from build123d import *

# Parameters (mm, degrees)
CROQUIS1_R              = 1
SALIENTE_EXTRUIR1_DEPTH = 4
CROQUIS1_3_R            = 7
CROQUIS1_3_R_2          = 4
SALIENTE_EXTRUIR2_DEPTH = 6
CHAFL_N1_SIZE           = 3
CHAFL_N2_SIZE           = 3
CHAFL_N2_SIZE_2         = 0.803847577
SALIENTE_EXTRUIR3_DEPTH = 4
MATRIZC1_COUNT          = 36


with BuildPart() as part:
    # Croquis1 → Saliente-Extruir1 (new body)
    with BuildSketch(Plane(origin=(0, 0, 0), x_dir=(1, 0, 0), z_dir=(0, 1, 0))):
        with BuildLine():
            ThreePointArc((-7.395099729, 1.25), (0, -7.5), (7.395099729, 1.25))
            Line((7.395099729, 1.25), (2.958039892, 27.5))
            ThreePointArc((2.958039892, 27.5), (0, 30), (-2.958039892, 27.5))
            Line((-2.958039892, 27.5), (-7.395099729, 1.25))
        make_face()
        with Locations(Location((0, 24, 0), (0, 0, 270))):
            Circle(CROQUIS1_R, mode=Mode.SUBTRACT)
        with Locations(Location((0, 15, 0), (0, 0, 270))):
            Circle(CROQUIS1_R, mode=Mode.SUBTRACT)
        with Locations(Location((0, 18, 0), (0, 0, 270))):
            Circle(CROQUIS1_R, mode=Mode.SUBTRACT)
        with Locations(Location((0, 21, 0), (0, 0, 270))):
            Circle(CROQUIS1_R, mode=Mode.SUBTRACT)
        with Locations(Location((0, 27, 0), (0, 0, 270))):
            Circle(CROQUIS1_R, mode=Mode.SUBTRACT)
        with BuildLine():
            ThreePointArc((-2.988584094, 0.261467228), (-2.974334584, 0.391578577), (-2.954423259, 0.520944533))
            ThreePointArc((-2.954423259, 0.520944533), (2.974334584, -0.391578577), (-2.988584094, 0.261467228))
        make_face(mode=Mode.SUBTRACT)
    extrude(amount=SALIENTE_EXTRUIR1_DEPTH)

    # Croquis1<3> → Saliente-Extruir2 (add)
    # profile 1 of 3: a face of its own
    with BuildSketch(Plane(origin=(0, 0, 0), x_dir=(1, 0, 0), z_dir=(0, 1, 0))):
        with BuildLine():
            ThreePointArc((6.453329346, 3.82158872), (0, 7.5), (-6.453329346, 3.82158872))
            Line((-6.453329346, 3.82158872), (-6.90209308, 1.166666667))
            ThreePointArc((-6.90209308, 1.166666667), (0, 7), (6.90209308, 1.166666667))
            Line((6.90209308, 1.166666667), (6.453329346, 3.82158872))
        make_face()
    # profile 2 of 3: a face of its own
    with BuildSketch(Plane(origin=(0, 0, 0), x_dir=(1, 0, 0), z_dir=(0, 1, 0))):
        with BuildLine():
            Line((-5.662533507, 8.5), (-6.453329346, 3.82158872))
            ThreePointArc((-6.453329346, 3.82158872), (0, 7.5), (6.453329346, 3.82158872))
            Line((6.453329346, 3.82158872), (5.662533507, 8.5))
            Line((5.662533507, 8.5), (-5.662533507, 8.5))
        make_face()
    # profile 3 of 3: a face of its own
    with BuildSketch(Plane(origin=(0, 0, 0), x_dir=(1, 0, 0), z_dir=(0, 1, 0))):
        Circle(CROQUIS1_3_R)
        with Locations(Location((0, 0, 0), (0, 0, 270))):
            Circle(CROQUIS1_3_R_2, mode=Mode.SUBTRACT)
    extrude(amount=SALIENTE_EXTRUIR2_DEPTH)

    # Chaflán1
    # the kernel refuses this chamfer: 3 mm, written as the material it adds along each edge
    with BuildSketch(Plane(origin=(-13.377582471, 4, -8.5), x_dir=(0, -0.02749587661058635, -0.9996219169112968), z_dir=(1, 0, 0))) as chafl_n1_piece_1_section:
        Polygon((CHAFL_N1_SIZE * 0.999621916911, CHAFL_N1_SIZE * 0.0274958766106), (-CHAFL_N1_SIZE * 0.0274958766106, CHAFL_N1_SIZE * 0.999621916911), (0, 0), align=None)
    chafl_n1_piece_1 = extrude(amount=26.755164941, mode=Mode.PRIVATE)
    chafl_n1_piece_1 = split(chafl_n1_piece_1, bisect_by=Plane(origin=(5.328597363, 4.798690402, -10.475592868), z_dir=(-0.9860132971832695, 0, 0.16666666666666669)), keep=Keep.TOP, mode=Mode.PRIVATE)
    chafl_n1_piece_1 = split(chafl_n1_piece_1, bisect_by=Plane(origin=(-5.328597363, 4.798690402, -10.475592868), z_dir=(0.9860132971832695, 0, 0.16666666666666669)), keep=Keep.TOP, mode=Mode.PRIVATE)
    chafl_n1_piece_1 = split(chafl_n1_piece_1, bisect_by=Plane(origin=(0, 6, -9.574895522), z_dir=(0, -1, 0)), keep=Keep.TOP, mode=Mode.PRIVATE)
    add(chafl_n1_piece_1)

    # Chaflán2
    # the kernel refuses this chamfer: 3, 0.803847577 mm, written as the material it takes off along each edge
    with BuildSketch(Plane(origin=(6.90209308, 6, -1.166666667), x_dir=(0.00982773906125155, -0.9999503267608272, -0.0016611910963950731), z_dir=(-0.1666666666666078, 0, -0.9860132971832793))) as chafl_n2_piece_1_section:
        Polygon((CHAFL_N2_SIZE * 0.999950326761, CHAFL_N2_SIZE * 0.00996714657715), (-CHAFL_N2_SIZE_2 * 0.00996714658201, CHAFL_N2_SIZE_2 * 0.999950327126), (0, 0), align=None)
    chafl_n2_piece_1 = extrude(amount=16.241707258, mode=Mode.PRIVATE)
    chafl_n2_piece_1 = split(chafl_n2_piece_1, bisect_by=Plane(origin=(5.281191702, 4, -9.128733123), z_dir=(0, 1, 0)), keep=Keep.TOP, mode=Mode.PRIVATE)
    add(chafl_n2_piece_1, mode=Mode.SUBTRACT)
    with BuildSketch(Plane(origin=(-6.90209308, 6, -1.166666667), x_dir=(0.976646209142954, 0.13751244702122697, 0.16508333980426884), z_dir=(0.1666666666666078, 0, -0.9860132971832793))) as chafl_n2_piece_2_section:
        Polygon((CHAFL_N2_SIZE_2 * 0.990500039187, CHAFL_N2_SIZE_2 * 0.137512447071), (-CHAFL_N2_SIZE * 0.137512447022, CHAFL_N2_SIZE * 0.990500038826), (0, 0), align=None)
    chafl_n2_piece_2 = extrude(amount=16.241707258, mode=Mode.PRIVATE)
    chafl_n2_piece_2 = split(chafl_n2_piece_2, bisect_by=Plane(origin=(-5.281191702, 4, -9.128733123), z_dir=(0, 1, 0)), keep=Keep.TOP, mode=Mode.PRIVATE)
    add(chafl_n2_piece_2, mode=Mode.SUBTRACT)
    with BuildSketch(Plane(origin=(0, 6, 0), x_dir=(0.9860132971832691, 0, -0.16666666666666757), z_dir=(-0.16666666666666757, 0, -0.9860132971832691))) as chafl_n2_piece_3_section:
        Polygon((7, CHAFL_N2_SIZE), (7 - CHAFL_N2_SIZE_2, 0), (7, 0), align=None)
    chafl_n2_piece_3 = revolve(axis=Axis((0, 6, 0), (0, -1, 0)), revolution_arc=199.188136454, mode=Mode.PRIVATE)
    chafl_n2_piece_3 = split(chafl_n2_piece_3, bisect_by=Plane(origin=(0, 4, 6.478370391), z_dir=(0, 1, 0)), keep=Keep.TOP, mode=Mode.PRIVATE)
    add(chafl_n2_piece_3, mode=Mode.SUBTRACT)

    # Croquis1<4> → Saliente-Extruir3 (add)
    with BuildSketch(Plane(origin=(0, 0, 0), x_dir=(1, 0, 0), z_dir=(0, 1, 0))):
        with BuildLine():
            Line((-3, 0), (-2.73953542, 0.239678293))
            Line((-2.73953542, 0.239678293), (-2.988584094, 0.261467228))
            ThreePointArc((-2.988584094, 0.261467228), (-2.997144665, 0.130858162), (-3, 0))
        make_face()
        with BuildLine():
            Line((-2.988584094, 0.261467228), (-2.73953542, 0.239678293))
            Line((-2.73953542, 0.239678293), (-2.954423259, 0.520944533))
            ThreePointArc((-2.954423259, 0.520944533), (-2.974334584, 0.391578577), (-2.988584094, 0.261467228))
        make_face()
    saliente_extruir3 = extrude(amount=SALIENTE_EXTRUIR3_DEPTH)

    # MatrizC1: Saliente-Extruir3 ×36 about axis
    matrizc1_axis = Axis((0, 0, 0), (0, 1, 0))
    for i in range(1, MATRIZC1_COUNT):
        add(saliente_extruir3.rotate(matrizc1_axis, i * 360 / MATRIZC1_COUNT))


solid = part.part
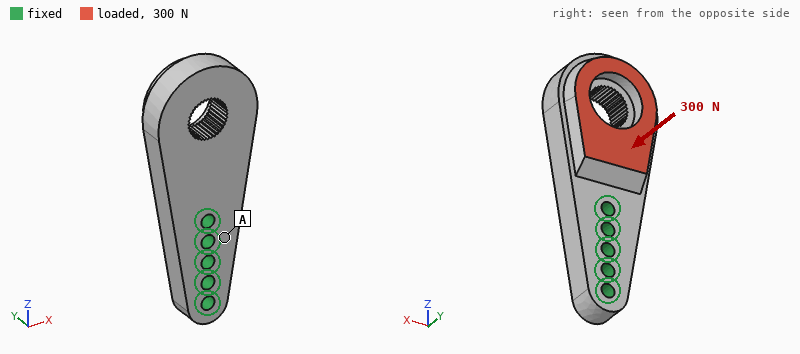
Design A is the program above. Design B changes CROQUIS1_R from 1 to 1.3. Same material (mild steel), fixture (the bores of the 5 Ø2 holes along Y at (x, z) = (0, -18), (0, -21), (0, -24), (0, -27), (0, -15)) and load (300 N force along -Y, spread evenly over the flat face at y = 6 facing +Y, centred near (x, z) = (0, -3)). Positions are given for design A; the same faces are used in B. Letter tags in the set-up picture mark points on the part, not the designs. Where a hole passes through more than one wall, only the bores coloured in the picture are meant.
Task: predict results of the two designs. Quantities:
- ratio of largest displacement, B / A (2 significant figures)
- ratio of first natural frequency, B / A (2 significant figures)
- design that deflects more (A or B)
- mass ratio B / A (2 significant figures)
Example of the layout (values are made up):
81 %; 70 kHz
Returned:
0.90; 1.1; A; 0.97
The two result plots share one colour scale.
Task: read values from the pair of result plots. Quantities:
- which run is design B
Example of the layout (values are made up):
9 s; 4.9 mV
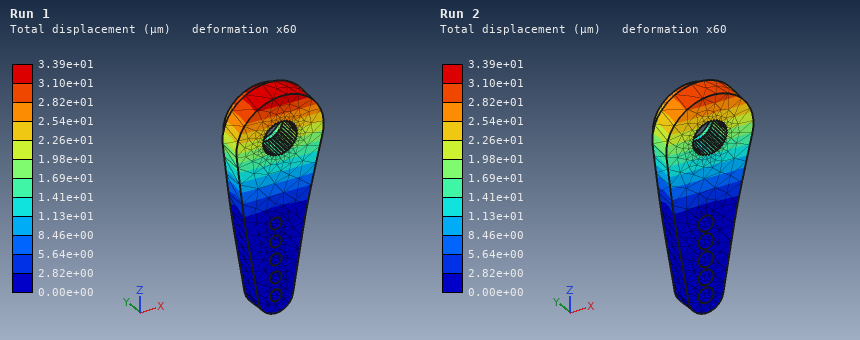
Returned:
Run 2
